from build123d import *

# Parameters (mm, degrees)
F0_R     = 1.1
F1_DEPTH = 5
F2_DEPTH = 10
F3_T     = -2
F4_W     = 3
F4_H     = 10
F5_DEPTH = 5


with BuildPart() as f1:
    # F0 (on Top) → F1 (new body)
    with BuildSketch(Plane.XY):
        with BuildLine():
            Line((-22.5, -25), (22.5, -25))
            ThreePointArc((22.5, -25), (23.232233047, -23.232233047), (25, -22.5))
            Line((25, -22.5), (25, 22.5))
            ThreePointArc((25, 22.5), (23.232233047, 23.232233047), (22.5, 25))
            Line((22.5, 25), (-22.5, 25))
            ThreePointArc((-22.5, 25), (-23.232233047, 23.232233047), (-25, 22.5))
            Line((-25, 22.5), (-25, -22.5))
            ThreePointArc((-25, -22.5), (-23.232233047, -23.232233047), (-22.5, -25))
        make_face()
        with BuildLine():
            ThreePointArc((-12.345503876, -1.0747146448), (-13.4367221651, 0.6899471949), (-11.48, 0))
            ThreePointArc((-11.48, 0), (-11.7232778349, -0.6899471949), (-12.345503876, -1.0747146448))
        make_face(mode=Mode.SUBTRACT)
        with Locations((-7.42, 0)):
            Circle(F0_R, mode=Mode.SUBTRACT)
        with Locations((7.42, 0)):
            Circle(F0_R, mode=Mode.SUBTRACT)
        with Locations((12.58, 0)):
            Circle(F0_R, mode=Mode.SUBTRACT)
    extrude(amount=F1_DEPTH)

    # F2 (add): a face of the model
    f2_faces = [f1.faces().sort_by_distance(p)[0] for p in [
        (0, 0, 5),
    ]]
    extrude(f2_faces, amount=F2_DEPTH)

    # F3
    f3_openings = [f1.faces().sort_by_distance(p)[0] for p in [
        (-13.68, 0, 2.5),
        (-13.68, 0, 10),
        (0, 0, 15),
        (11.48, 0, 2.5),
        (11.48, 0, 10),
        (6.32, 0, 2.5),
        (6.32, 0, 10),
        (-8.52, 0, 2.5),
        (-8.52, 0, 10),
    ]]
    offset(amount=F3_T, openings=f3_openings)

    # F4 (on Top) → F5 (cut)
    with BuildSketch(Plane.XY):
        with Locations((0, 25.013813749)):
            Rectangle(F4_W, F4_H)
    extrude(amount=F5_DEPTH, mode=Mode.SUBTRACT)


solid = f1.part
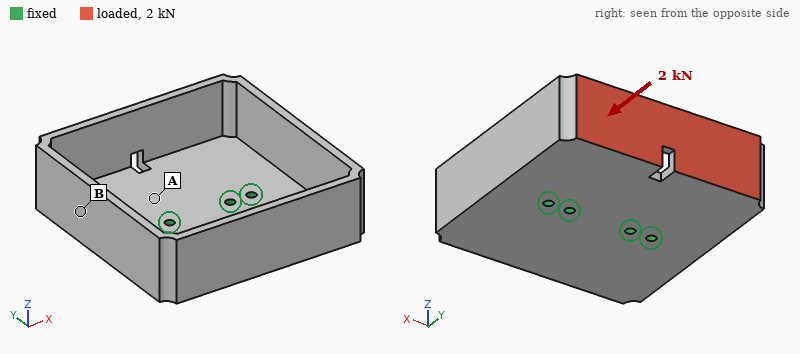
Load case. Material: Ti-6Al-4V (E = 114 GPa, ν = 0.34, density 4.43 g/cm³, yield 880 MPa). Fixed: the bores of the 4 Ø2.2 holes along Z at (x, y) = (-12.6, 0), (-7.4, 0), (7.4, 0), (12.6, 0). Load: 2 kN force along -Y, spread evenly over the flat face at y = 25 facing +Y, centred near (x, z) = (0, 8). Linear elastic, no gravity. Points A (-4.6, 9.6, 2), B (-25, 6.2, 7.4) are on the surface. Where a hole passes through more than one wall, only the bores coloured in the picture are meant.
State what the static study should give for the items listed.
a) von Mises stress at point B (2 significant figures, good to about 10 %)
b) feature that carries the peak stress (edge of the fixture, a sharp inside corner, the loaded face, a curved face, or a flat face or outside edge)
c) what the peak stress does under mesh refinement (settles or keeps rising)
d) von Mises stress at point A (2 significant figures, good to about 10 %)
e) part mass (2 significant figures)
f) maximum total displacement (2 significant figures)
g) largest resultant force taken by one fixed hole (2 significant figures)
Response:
50 MPa
edge of the fixture
keeps rising
140 MPa
43 g
0.60 mm
630 N
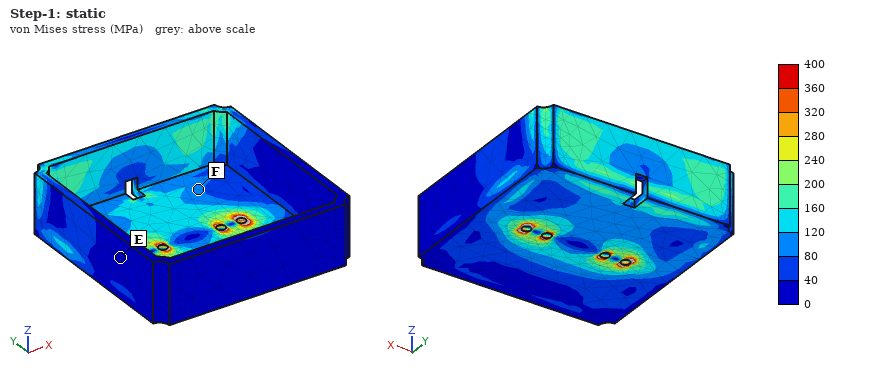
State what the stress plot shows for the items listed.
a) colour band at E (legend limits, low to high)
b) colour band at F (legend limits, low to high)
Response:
0 to 40 MPa
80 to 120 MPa
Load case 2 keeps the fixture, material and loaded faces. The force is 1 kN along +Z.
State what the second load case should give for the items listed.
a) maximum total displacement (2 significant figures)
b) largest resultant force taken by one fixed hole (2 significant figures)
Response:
0.80 mm
560 N
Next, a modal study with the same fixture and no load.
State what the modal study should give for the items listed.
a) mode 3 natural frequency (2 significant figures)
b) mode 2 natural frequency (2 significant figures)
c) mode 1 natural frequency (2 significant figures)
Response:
3000 Hz
2200 Hz
1400 Hz
